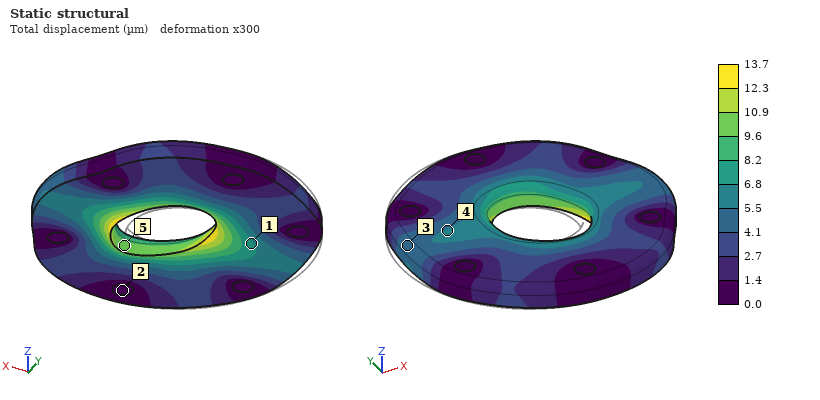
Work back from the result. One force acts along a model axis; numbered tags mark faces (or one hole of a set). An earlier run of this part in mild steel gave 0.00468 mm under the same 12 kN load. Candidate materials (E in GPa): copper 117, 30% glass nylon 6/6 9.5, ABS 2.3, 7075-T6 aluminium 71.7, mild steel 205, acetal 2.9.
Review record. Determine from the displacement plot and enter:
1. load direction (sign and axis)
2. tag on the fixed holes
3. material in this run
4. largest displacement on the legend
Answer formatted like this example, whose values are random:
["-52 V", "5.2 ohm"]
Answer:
["+X", "2", "7075-T6 aluminium", "13.7 µm"]
